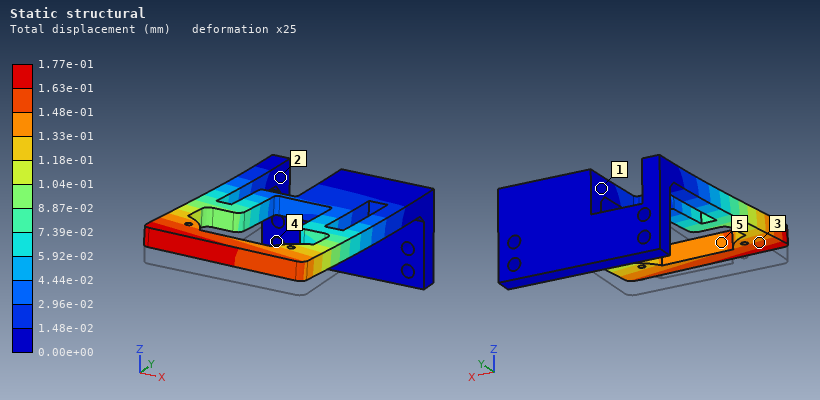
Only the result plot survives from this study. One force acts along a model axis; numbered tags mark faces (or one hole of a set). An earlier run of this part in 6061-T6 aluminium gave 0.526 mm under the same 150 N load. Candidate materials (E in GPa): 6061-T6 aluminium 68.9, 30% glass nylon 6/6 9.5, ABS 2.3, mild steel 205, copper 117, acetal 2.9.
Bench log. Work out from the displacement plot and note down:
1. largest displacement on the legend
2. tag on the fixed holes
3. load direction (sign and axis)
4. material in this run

1.77e-01 mm
4
+Z
mild steel
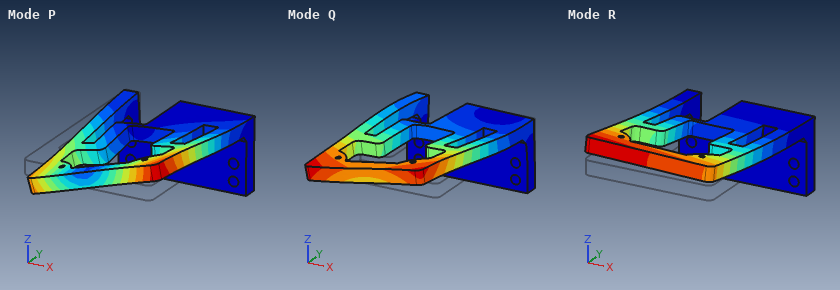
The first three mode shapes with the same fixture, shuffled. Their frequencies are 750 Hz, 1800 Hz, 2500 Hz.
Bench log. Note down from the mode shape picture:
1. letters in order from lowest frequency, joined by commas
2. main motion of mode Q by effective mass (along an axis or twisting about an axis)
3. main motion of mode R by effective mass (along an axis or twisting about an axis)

R, P, Q
along X
along Z
